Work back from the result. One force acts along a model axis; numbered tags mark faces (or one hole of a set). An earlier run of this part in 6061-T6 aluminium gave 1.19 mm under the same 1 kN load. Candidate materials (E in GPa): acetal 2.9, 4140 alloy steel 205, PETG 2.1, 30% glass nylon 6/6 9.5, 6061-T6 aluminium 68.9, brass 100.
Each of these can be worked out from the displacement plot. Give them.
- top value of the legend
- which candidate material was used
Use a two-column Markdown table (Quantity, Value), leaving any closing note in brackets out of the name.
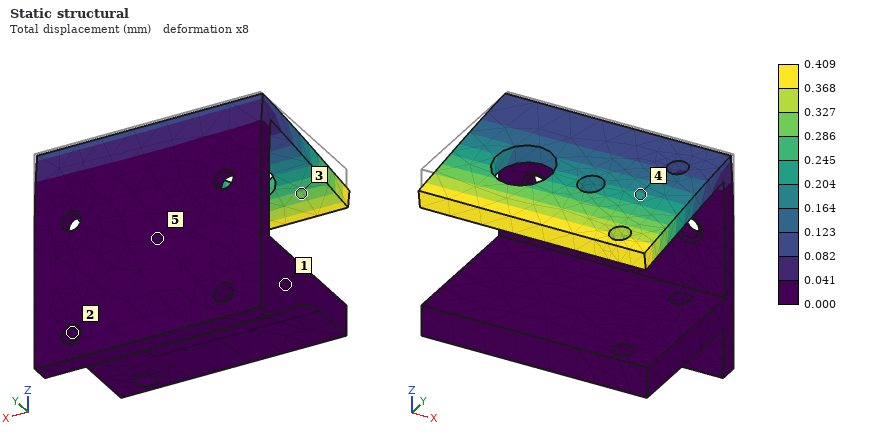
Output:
| Quantity | Value |
|---|---|
| top value of the legend | 0.409 mm |
| which candidate material was used | 4140 alloy steel |
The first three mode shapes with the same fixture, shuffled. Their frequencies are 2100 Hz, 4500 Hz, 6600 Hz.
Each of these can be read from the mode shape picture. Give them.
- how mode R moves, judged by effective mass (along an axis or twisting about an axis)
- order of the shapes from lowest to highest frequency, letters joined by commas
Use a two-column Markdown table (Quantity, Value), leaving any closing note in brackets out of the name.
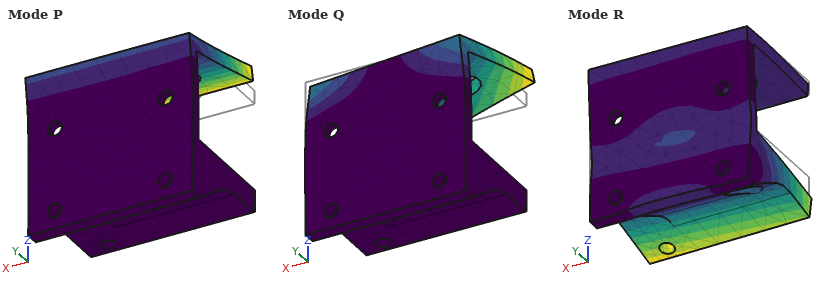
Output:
| Quantity | Value |
|---|---|
| how mode R moves, judged by effective mass | along Z |
| order of the shapes from lowest to highest frequency, letters joined by commas | P, Q, R |
